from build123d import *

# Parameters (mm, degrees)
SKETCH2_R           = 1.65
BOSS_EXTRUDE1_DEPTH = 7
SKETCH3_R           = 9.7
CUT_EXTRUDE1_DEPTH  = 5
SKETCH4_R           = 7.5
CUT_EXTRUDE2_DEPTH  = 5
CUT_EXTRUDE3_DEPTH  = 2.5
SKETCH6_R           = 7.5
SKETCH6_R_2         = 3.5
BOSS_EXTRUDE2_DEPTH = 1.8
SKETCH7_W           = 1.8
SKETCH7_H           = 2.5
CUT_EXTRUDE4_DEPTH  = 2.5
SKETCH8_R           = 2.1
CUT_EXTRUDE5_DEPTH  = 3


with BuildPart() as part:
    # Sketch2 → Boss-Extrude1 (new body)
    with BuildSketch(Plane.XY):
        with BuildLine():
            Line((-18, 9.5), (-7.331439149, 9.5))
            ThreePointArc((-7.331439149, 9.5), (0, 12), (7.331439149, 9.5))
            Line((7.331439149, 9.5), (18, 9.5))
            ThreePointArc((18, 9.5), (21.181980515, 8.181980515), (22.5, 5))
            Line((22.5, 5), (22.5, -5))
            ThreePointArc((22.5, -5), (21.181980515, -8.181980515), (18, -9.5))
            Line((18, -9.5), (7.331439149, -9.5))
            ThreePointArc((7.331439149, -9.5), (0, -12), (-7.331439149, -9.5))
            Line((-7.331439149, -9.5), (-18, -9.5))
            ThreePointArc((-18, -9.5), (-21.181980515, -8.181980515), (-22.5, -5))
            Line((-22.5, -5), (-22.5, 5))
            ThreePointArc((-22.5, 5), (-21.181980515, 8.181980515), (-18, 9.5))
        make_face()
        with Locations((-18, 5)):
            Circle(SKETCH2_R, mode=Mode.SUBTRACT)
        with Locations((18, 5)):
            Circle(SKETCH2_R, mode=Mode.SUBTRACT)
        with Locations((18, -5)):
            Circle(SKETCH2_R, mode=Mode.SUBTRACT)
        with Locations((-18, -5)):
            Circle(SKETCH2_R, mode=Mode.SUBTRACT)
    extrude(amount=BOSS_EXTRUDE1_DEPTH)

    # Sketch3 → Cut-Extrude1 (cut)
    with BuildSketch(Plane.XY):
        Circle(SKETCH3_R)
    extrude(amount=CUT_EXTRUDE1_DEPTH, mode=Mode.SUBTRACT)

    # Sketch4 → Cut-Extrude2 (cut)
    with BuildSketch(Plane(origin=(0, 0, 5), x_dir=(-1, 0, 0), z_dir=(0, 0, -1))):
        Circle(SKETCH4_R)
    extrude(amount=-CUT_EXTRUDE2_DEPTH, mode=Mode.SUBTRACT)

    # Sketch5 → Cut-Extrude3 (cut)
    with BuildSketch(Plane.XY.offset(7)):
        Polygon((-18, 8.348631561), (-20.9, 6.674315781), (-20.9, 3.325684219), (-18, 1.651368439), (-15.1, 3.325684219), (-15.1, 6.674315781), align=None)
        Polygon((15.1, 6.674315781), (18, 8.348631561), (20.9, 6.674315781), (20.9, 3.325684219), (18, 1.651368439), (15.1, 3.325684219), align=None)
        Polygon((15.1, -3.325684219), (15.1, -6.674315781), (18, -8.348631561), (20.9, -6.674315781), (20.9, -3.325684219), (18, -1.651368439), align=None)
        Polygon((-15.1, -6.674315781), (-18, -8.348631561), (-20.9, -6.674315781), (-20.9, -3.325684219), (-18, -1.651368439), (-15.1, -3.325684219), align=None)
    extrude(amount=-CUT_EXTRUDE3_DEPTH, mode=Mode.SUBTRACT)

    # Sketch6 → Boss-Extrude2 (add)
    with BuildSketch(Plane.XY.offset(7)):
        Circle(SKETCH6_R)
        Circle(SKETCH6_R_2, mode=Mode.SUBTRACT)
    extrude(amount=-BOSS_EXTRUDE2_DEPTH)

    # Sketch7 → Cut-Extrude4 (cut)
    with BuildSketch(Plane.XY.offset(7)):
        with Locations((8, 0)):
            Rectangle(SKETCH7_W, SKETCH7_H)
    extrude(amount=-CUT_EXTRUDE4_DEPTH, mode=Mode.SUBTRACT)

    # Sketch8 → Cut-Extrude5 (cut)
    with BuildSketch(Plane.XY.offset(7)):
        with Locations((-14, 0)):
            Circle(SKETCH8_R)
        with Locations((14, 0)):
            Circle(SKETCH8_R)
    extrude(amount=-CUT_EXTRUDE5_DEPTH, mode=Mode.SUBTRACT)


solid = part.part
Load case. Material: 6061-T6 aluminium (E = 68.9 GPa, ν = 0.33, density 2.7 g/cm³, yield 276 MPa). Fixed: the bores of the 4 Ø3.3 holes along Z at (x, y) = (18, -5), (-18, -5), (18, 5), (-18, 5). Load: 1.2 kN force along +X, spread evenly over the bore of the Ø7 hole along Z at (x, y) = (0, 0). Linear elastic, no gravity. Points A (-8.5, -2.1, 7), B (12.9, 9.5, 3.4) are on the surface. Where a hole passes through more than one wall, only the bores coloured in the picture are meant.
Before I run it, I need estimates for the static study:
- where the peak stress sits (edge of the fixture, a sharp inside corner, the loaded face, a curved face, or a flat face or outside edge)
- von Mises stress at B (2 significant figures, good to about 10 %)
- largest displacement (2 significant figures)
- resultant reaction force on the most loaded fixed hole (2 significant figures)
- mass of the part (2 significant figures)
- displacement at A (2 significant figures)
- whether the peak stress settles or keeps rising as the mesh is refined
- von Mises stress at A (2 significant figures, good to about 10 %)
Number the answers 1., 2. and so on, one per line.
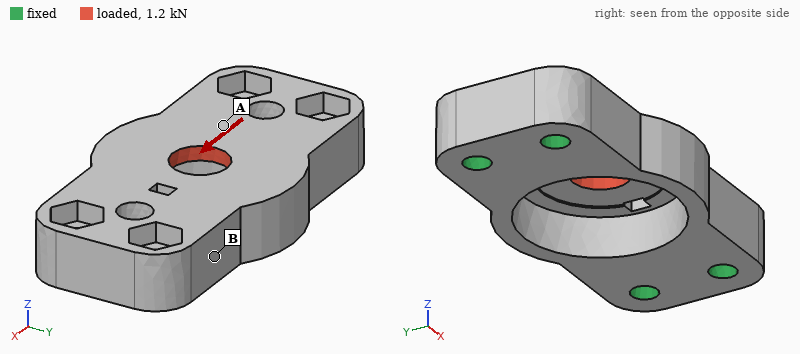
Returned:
1. a sharp inside corner
2. 6.3 MPa
3. 5.7 µm
4. 310 N
5. 11 g
6. 3.6 µm
7. keeps rising
8. 21 MPa
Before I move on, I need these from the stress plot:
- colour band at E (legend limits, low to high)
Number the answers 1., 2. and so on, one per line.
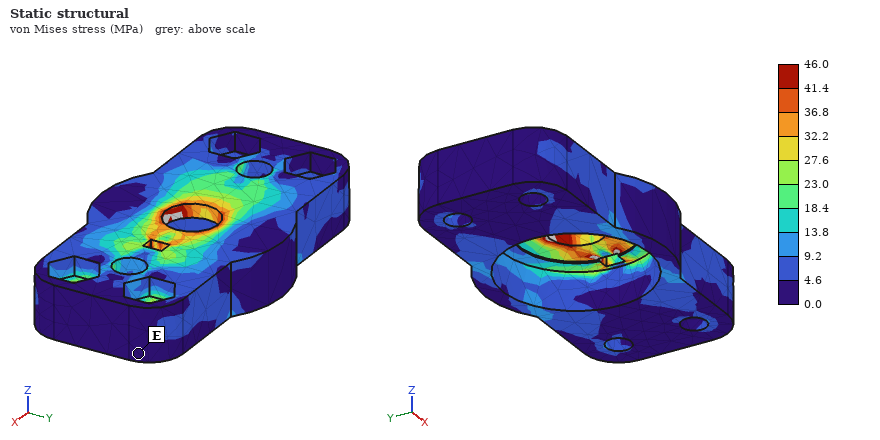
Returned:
1. 0.0 to 4.6 MPa
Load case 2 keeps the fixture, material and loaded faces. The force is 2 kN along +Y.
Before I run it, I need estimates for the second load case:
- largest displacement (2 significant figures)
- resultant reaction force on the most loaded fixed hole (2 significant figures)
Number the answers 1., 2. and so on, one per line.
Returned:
1. 18 µm
2. 830 N
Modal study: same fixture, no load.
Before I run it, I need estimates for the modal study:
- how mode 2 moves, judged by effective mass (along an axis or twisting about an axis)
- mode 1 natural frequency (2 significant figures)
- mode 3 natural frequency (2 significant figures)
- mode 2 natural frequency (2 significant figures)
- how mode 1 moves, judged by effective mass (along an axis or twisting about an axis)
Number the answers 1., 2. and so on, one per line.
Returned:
1. twisting about X
2. 22 kHz
3. 39 kHz
4. 24 kHz
5. along Z
